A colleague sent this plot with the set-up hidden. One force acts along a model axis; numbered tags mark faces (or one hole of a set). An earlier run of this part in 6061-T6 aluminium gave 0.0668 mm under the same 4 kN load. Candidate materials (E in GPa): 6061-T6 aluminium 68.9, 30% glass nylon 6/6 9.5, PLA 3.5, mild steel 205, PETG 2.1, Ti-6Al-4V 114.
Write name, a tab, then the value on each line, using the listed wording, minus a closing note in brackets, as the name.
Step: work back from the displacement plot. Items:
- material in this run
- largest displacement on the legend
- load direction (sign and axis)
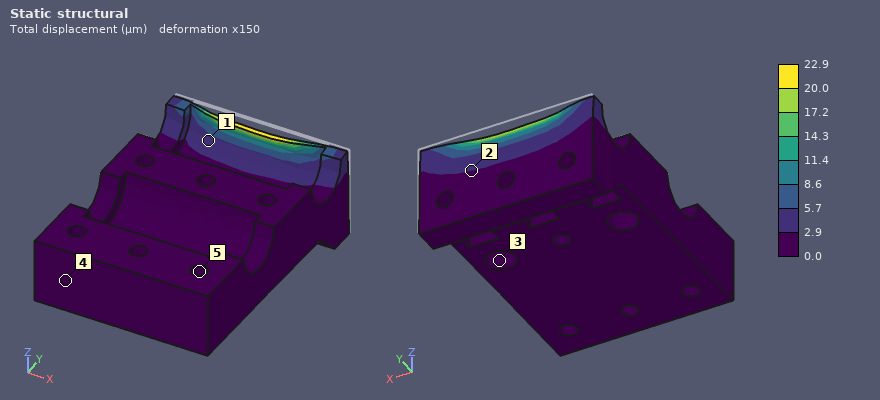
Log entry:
material in this run	mild steel
largest displacement on the legend	22.9 µm
load direction	-Y
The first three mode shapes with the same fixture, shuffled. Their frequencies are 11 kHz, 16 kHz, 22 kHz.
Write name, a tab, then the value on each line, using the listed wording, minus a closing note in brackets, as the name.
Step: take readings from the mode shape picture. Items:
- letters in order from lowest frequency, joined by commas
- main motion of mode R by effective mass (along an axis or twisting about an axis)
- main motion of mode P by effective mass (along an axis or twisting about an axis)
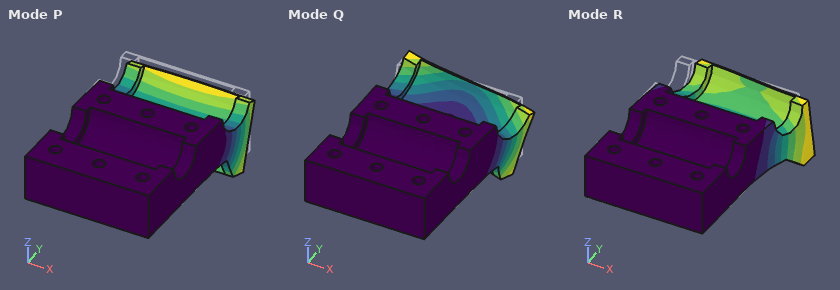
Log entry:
letters in order from lowest frequency, joined by commas	P, Q, R
main motion of mode R by effective mass	along X
main motion of mode P by effective mass	along Z
